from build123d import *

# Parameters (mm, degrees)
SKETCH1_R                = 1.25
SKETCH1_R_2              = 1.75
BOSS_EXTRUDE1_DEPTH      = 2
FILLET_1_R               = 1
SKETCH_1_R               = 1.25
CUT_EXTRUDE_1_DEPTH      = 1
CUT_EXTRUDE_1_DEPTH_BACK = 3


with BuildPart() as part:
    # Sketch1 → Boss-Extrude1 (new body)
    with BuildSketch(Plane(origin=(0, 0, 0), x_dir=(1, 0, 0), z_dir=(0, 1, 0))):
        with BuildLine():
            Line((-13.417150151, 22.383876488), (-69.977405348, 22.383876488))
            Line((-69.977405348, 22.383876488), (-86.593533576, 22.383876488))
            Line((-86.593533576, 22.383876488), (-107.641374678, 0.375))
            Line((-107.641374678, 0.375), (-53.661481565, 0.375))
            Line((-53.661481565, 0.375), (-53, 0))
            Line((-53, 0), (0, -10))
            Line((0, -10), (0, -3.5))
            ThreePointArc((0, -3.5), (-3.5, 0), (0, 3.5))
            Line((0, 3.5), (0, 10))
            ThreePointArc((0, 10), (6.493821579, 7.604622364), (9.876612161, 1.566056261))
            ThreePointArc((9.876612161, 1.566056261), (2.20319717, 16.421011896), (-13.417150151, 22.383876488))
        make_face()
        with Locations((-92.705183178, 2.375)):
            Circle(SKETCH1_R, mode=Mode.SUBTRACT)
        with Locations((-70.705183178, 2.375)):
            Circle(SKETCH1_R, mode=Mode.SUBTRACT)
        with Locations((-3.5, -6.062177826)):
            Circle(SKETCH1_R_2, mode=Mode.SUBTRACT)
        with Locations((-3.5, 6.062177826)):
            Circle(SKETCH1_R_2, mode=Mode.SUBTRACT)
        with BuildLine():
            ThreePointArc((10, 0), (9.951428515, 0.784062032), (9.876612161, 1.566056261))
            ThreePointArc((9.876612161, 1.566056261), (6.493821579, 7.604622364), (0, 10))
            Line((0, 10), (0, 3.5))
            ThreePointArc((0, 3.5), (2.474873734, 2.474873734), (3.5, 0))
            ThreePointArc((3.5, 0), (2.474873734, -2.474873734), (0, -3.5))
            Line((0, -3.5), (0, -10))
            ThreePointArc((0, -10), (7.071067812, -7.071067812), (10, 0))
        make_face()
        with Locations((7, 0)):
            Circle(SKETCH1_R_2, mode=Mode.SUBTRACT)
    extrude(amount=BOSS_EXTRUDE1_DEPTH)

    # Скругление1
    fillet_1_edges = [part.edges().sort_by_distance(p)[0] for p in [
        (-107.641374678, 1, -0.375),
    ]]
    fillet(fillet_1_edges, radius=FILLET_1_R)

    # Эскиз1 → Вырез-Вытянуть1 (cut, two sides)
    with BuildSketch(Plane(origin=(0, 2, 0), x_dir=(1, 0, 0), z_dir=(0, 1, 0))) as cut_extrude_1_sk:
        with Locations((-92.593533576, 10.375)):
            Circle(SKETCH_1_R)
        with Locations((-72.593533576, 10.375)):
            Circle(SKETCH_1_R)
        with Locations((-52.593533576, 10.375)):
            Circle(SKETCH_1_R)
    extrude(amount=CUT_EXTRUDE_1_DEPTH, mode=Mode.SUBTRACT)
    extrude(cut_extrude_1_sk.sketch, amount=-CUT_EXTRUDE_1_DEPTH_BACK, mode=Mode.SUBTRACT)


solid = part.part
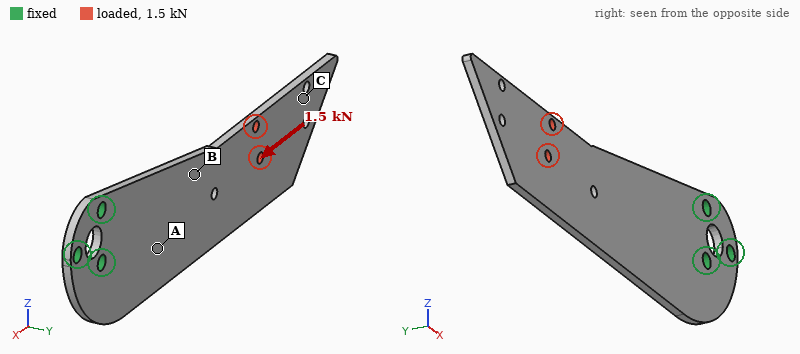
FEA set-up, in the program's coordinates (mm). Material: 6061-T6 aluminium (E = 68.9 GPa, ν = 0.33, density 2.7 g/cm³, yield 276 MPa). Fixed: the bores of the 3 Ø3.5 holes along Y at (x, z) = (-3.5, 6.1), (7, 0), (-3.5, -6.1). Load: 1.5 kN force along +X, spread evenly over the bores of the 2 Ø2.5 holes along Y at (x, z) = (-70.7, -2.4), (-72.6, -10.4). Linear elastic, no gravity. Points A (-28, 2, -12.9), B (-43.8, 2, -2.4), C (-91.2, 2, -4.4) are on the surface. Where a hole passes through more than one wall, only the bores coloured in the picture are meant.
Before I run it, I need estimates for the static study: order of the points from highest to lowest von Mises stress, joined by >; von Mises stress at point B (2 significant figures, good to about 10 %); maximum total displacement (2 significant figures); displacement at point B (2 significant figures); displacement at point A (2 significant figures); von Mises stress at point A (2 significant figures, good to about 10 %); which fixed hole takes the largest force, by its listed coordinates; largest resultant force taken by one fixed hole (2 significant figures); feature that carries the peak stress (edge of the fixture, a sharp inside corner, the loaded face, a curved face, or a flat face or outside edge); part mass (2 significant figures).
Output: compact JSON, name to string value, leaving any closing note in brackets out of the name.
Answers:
{"order of the points from highest to lowest von Mises stress, joined by >": "B > A > C", "von Mises stress at point B": "52 MPa", "maximum total displacement": "89 µm", "displacement at point B": "26 µm", "displacement at point A": "20 µm", "von Mises stress at point A": "25 MPa", "which fixed hole takes the largest force, by its listed coordinates": "(-3.5, -6.1)", "largest resultant force taken by one fixed hole": "1.2 kN", "feature that carries the peak stress": "the loaded face", "part mass": "14 g"}
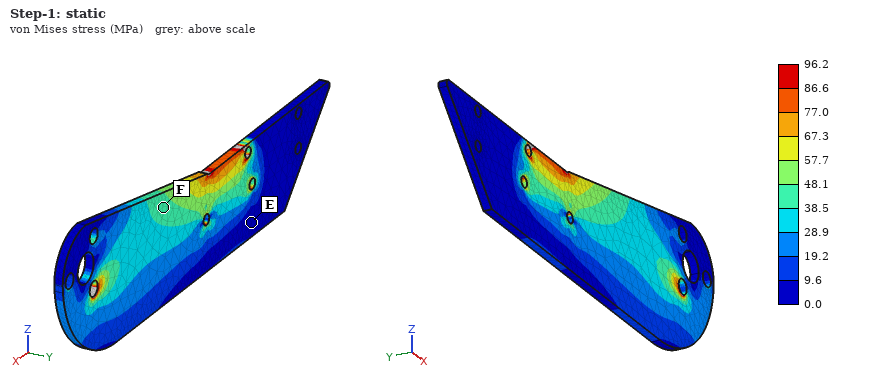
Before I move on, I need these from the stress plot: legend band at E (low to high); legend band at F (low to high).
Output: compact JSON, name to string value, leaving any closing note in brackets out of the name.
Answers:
{"legend band at E": "0.0 to 9.6 MPa", "legend band at F": "38.5 to 48.1 MPa"}
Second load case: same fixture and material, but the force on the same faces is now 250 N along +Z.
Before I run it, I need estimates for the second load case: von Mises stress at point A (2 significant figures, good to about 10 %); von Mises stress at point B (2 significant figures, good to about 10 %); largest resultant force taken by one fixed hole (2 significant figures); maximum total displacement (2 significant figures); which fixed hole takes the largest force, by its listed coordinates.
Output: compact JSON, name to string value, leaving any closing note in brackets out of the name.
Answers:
{"von Mises stress at point A": "15 MPa", "von Mises stress at point B": "26 MPa", "largest resultant force taken by one fixed hole": "1.0 kN", "maximum total displacement": "0.29 mm", "which fixed hole takes the largest force, by its listed coordinates": "(-3.5, 6.1)"}
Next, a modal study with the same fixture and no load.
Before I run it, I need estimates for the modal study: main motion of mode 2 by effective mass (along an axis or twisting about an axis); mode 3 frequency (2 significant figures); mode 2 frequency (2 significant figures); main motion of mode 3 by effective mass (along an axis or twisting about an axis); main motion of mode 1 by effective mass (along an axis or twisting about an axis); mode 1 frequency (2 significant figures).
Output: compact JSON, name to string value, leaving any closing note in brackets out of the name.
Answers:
{"main motion of mode 2 by effective mass": "along Y", "mode 3 frequency": "1700 Hz", "mode 2 frequency": "1100 Hz", "main motion of mode 3 by effective mass": "twisting about X", "main motion of mode 1 by effective mass": "along Y", "mode 1 frequency": "210 Hz"}
